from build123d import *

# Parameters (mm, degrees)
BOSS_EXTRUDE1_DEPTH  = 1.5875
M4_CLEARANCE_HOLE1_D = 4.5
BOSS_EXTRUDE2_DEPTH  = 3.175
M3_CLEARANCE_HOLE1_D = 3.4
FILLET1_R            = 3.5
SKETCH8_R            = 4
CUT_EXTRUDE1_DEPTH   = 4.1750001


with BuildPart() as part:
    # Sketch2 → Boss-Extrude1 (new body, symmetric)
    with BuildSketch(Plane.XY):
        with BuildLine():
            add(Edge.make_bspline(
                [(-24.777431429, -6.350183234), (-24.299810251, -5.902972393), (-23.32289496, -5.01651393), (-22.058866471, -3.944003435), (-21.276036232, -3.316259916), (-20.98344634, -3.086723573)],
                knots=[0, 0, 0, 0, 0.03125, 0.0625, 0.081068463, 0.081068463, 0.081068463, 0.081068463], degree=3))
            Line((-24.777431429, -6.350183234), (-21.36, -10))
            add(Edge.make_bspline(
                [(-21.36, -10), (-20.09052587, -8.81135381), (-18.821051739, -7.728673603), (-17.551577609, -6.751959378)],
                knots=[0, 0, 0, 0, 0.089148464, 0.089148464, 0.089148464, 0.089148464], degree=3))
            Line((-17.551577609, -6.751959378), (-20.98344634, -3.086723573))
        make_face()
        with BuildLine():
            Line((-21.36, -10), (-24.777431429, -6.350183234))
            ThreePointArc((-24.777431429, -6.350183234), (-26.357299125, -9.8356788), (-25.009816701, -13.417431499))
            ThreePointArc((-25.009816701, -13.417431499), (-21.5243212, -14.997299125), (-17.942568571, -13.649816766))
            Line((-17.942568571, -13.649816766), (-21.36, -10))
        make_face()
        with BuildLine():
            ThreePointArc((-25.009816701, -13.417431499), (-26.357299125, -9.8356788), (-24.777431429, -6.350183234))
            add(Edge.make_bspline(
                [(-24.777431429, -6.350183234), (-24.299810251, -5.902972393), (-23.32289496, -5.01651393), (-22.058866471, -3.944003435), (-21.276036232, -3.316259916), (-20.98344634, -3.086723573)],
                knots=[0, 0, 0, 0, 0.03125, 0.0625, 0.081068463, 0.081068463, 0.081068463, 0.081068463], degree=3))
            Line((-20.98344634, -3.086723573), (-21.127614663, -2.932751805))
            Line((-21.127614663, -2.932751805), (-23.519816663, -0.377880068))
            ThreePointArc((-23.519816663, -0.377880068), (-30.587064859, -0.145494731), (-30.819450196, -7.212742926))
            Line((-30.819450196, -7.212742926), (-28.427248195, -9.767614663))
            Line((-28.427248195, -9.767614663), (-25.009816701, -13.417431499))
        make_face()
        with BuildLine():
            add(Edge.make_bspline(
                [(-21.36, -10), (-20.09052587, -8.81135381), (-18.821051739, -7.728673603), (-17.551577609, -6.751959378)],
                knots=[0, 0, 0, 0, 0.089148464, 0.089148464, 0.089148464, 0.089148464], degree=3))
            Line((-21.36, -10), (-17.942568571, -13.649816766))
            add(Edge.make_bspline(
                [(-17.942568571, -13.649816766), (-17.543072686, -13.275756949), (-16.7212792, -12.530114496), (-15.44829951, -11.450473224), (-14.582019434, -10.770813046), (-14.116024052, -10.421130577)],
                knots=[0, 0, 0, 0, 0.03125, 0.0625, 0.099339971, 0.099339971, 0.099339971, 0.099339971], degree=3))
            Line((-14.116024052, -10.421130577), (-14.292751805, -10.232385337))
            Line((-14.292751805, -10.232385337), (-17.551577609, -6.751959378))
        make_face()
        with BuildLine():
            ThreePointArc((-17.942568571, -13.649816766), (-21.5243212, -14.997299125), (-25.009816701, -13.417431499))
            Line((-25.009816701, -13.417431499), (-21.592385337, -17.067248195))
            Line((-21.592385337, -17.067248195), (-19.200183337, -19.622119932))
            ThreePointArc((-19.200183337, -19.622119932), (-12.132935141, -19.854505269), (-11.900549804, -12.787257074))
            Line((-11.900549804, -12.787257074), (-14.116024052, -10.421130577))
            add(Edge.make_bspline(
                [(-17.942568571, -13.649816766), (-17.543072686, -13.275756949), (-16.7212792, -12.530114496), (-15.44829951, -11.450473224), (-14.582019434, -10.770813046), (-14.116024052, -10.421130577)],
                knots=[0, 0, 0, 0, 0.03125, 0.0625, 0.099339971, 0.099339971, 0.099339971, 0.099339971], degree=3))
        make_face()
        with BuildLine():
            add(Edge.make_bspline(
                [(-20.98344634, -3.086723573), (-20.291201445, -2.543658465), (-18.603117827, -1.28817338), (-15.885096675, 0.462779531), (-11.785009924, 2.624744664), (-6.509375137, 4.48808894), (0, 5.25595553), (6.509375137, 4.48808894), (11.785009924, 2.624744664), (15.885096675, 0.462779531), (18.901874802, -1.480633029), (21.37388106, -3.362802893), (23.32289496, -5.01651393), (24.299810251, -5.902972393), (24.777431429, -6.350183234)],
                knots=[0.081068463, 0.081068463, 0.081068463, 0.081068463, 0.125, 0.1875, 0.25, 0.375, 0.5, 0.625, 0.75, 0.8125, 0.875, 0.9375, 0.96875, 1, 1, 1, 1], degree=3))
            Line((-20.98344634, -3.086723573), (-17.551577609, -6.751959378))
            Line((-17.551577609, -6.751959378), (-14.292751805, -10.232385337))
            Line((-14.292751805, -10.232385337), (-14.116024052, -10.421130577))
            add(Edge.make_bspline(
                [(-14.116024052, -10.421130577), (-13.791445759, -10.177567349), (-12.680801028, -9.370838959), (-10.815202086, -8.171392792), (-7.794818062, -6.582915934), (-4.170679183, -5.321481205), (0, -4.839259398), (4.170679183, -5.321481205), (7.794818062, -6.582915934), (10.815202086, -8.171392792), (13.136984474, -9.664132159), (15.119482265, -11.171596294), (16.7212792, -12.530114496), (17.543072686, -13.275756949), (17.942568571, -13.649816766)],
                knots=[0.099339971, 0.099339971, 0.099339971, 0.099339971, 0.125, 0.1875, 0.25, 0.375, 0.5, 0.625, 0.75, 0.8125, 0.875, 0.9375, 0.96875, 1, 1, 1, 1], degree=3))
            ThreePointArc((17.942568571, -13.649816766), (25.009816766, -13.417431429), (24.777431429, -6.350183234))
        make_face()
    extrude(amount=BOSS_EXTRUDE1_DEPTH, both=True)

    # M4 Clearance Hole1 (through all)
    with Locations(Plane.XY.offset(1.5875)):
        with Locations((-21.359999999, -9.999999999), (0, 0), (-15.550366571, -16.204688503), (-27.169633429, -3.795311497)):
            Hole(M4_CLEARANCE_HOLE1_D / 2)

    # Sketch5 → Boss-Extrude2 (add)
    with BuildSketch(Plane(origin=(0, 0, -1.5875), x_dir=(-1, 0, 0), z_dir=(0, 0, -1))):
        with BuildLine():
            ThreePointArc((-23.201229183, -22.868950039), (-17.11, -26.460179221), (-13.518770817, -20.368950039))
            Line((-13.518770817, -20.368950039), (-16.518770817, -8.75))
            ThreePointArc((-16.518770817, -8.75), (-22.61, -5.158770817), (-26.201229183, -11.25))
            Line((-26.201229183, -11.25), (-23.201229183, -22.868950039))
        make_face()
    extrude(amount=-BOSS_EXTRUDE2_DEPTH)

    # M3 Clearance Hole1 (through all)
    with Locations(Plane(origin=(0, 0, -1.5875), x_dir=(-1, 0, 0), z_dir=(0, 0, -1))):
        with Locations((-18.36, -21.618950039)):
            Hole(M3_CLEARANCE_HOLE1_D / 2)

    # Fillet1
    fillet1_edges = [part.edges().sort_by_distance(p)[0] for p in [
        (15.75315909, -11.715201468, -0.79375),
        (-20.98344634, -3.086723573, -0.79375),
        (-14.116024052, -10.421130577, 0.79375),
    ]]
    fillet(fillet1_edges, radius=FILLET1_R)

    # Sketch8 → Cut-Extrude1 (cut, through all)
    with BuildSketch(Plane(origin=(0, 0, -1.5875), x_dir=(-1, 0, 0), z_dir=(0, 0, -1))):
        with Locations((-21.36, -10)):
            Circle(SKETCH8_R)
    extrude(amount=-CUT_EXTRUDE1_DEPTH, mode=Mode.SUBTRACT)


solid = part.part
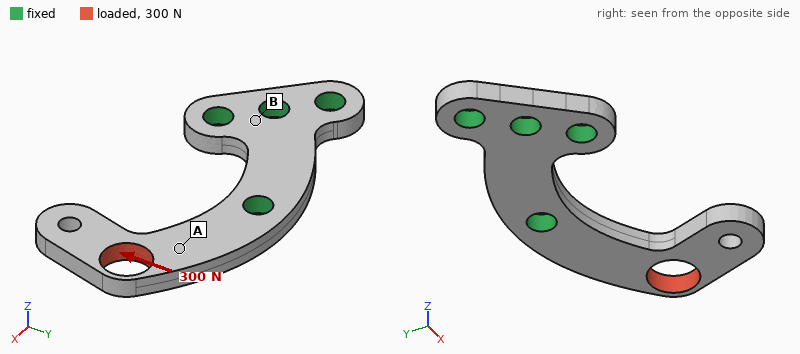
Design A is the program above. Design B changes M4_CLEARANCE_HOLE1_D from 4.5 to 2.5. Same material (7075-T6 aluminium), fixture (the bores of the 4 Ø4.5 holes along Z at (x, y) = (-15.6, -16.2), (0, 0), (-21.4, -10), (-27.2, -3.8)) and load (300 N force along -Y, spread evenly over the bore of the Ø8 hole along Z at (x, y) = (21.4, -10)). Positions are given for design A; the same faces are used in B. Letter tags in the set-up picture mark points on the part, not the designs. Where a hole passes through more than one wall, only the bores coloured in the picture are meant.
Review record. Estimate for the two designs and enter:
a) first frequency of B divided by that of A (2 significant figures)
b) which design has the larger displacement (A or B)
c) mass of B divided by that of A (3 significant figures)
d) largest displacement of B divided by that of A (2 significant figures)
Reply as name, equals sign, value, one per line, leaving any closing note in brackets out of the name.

first frequency of B divided by that of A = 0.94
which design has the larger displacement = B
mass of B divided by that of A = 1.06
largest displacement of B divided by that of A = 1.2
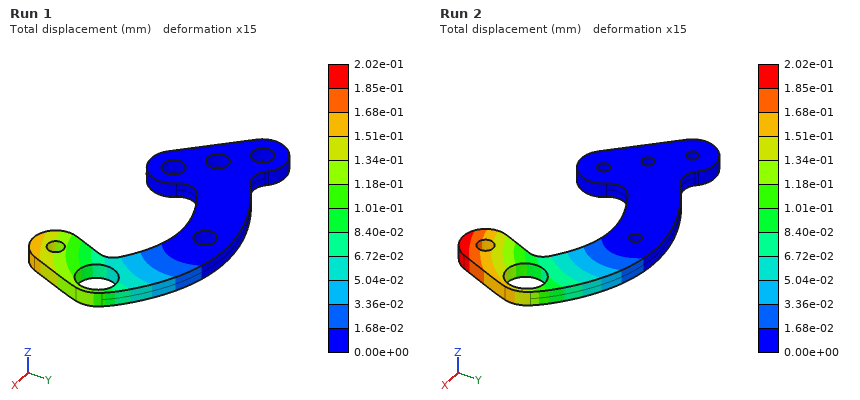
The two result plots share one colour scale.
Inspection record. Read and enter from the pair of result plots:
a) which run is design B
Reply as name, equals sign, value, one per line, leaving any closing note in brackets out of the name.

which run is design B = Run 2
